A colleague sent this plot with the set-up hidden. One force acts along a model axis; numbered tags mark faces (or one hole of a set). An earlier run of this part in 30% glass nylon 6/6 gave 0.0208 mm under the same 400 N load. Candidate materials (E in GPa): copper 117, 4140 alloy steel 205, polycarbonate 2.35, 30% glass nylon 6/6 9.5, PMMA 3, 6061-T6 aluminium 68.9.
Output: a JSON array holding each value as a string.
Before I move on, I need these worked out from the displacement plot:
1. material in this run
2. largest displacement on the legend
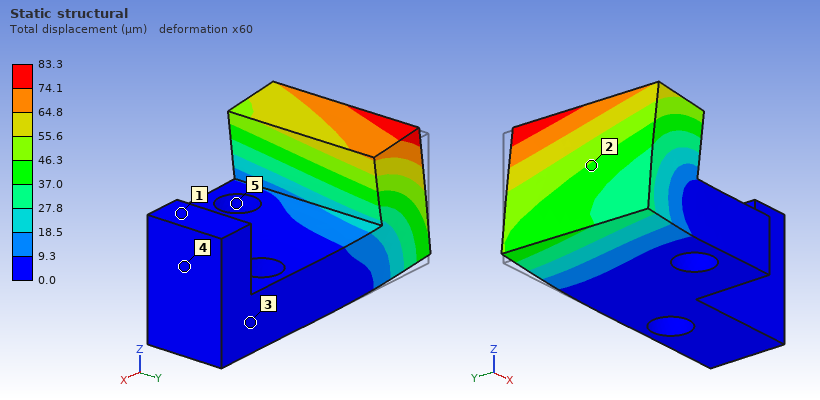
["polycarbonate", "83.3 µm"]
